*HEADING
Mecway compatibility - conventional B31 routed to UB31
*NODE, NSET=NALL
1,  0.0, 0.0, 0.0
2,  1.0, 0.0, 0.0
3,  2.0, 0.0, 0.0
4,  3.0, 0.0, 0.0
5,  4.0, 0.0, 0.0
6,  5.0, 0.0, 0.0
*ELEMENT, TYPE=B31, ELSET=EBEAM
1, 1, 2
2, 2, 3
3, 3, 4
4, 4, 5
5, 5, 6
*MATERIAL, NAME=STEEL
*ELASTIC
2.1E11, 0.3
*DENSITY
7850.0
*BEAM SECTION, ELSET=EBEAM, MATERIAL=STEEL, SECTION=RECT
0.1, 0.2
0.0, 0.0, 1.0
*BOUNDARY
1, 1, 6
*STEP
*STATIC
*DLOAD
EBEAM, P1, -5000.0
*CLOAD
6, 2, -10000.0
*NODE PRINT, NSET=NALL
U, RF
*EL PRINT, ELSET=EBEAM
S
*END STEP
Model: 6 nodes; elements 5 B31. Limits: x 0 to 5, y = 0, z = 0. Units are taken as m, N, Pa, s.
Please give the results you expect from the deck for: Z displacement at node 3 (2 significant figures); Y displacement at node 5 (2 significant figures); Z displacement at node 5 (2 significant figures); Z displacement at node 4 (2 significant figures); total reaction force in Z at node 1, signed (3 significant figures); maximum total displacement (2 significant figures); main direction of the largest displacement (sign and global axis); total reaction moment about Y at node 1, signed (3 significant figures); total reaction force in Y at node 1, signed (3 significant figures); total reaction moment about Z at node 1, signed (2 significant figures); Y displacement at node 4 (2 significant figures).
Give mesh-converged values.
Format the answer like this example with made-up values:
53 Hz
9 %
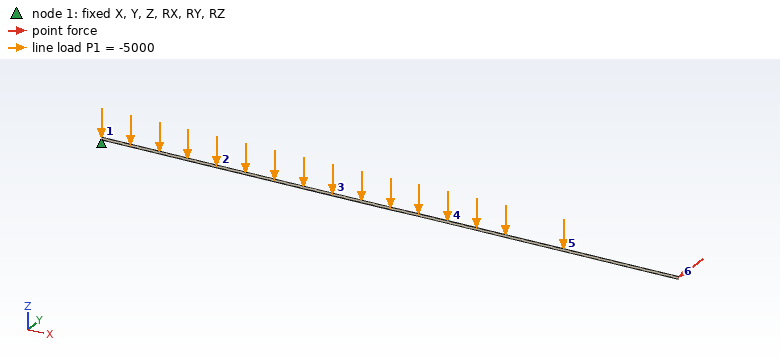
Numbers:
-0.027 m
-0.021 m
-0.082 m
-0.053 m
25000 N
0.12 m
-Z
-62500 N·m
10000 N
50000 N·m
-0.013 m
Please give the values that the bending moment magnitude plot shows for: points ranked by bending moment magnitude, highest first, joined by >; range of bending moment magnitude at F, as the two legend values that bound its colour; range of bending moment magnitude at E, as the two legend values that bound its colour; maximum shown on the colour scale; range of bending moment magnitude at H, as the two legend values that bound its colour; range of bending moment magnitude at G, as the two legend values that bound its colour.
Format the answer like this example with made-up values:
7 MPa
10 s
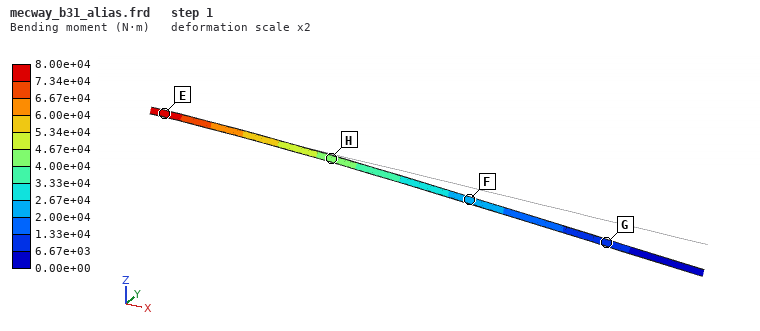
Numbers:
E > H > F > G
2.00e+04 to 2.67e+04 N·m
7.34e+04 to 8.00e+04 N·m
8.00e+04 N·m
4.00e+04 to 4.67e+04 N·m
6.67e+03 to 1.33e+04 N·m
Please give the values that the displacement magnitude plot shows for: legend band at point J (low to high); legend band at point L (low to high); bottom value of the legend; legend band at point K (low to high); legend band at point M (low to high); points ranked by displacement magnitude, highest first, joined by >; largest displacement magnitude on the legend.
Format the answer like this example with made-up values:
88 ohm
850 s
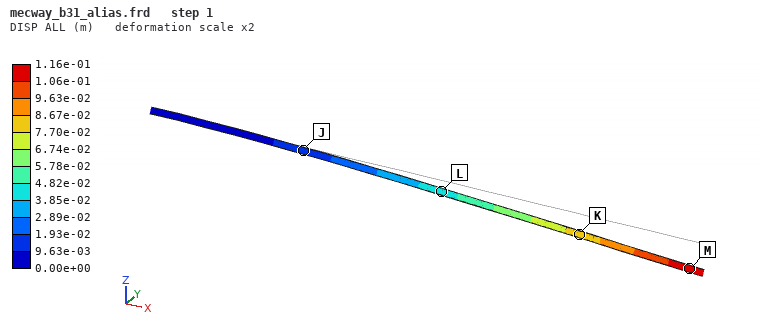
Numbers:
9.63e-03 to 1.93e-02 m
3.85e-02 to 4.82e-02 m
0.00e+00 m
7.70e-02 to 8.67e-02 m
1.06e-01 to 1.16e-01 m
M > K > L > J
1.16e-01 m
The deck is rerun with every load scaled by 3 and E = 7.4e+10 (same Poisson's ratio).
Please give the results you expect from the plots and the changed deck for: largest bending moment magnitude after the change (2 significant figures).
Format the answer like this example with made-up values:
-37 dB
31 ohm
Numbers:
2.4e+05 N·m
